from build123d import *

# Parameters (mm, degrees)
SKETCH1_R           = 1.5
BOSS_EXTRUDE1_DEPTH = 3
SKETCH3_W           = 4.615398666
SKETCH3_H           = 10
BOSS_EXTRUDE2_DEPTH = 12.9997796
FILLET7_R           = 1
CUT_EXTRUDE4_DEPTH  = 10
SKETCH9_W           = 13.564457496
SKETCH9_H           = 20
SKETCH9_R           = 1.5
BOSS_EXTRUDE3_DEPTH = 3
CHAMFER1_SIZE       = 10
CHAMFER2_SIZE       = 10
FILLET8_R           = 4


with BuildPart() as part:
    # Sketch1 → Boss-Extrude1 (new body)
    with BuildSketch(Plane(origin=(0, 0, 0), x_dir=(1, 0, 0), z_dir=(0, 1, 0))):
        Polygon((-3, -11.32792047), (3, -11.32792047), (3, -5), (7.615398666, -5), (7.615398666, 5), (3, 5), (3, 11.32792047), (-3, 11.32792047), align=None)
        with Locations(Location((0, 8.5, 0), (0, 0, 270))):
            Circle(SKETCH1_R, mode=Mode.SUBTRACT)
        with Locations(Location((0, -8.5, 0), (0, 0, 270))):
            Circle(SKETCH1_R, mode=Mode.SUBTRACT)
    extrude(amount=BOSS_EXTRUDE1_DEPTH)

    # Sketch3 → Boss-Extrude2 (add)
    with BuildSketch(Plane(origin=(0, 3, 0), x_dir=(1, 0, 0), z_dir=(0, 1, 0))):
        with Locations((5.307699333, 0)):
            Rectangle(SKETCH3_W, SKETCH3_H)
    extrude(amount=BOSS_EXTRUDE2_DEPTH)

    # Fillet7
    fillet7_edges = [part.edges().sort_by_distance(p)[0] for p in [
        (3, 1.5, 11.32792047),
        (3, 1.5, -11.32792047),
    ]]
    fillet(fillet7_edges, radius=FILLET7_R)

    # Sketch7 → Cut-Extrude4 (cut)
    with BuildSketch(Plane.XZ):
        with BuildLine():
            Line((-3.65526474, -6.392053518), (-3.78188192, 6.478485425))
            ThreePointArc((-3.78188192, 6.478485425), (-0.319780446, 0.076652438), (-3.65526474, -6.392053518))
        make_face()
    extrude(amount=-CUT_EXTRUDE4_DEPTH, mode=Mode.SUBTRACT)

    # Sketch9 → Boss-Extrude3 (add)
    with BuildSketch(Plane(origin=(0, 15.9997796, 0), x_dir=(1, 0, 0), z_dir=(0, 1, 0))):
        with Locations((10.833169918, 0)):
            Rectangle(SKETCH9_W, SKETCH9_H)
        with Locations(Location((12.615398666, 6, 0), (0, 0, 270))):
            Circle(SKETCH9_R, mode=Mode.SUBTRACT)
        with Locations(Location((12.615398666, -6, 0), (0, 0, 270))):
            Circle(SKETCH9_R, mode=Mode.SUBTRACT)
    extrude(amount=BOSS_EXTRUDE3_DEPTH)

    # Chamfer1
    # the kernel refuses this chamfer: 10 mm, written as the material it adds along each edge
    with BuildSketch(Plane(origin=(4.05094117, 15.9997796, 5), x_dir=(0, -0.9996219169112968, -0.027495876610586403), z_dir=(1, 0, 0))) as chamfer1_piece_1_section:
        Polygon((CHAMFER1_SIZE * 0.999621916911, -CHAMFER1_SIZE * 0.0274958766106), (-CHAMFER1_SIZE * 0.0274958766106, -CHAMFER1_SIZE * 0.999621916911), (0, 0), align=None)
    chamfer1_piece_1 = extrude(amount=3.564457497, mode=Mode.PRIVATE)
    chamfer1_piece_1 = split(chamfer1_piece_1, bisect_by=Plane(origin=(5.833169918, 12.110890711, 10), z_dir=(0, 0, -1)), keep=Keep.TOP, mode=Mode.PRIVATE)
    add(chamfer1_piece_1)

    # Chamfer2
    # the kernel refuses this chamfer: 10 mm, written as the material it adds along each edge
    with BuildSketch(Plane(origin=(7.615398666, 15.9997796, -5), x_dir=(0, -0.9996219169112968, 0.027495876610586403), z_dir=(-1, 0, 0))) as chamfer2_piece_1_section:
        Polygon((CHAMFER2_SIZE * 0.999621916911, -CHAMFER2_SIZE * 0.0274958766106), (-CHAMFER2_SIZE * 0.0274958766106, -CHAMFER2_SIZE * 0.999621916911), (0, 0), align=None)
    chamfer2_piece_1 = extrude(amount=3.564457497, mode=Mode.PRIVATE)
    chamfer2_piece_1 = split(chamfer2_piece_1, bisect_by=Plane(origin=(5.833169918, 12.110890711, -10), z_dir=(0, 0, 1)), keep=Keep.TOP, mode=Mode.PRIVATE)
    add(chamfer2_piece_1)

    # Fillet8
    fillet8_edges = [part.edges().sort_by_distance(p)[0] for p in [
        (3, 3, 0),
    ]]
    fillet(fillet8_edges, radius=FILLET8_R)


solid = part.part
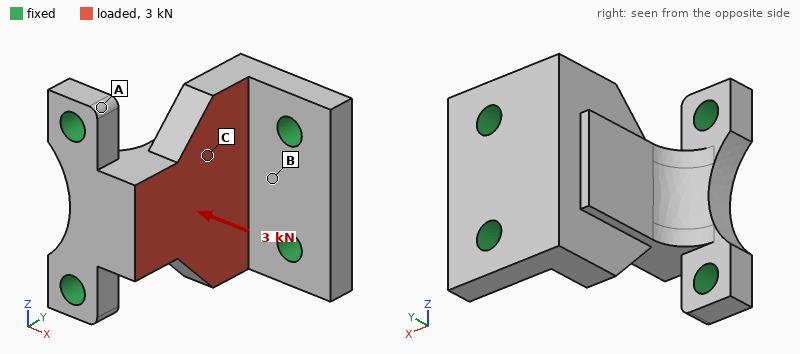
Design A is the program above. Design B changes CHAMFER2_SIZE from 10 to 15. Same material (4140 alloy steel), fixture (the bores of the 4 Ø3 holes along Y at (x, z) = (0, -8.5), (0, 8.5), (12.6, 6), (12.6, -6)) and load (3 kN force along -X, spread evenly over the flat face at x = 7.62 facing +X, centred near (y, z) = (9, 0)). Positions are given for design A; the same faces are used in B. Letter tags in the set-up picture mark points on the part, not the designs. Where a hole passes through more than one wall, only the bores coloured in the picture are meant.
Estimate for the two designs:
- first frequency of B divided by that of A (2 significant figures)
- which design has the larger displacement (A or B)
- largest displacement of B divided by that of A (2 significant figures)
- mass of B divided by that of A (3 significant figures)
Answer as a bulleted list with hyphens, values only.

- 0.98
- B
- 1.1
- 1.04
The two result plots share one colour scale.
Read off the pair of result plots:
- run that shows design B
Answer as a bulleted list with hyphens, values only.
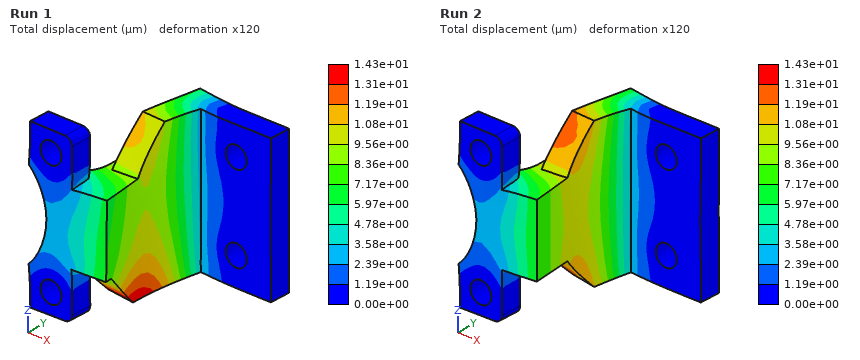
- Run 1
